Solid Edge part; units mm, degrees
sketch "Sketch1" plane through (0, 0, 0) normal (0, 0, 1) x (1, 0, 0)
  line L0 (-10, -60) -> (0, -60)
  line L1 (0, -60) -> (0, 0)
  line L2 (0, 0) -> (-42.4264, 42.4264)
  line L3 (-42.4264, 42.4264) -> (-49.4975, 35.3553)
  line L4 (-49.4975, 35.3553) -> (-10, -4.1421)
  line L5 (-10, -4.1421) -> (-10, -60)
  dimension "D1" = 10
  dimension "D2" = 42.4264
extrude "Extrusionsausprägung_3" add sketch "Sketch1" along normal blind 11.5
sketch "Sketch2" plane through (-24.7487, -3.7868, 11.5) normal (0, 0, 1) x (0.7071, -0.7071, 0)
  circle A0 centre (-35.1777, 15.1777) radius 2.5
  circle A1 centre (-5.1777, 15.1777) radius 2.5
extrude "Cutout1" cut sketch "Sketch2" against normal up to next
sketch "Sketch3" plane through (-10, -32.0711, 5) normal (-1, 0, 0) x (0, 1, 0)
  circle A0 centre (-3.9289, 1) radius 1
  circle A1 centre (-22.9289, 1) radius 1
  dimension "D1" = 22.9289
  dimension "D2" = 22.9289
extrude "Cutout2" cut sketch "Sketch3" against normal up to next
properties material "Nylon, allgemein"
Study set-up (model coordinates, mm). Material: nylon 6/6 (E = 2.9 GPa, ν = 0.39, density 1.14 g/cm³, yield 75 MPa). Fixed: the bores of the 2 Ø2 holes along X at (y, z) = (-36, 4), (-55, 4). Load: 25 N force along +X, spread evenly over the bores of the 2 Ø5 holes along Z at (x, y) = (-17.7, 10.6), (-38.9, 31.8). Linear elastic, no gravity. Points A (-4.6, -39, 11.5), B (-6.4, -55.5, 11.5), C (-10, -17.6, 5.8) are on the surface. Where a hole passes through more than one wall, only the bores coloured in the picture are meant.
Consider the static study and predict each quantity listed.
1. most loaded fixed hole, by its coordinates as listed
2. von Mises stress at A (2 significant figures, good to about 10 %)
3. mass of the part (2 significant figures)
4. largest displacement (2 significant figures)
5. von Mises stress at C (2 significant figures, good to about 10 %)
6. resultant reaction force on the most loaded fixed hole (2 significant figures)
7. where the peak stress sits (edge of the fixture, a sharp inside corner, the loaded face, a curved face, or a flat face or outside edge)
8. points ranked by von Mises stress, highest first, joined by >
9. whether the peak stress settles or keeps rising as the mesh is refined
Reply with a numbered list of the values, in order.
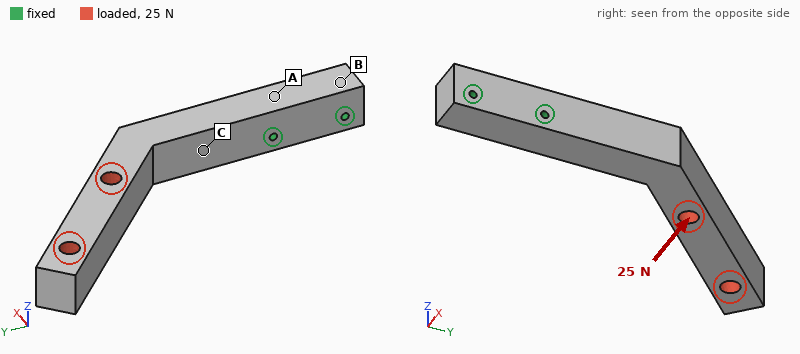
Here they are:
1. (-36, 4)
2. 1.5 MPa
3. 15 g
4. 1.2 mm
5. 5.1 MPa
6. 47 N
7. edge of the fixture
8. C > A > B
9. keeps rising
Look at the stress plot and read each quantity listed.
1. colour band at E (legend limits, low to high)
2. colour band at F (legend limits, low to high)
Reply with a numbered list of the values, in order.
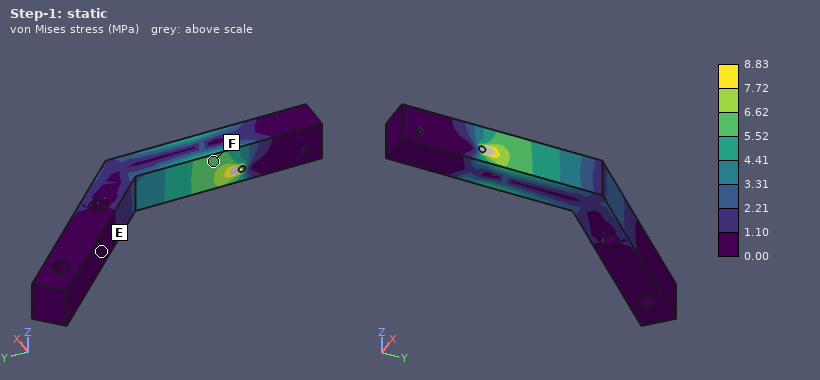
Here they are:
1. 0.00 to 1.10 MPa
2. 5.52 to 6.62 MPa
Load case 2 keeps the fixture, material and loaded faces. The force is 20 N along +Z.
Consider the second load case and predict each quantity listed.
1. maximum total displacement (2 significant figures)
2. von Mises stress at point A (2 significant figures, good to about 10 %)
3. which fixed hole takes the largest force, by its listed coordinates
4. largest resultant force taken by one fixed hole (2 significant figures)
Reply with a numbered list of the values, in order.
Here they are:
1. 1.1 mm
2. 3.8 MPa
3. (-36, 4)
4. 83 N
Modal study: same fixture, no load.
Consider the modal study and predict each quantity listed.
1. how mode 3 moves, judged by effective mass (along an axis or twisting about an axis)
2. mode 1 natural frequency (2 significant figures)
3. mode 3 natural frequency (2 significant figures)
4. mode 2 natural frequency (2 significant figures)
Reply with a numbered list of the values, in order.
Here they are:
1. along Z
2. 320 Hz
3. 1400 Hz
4. 320 Hz
